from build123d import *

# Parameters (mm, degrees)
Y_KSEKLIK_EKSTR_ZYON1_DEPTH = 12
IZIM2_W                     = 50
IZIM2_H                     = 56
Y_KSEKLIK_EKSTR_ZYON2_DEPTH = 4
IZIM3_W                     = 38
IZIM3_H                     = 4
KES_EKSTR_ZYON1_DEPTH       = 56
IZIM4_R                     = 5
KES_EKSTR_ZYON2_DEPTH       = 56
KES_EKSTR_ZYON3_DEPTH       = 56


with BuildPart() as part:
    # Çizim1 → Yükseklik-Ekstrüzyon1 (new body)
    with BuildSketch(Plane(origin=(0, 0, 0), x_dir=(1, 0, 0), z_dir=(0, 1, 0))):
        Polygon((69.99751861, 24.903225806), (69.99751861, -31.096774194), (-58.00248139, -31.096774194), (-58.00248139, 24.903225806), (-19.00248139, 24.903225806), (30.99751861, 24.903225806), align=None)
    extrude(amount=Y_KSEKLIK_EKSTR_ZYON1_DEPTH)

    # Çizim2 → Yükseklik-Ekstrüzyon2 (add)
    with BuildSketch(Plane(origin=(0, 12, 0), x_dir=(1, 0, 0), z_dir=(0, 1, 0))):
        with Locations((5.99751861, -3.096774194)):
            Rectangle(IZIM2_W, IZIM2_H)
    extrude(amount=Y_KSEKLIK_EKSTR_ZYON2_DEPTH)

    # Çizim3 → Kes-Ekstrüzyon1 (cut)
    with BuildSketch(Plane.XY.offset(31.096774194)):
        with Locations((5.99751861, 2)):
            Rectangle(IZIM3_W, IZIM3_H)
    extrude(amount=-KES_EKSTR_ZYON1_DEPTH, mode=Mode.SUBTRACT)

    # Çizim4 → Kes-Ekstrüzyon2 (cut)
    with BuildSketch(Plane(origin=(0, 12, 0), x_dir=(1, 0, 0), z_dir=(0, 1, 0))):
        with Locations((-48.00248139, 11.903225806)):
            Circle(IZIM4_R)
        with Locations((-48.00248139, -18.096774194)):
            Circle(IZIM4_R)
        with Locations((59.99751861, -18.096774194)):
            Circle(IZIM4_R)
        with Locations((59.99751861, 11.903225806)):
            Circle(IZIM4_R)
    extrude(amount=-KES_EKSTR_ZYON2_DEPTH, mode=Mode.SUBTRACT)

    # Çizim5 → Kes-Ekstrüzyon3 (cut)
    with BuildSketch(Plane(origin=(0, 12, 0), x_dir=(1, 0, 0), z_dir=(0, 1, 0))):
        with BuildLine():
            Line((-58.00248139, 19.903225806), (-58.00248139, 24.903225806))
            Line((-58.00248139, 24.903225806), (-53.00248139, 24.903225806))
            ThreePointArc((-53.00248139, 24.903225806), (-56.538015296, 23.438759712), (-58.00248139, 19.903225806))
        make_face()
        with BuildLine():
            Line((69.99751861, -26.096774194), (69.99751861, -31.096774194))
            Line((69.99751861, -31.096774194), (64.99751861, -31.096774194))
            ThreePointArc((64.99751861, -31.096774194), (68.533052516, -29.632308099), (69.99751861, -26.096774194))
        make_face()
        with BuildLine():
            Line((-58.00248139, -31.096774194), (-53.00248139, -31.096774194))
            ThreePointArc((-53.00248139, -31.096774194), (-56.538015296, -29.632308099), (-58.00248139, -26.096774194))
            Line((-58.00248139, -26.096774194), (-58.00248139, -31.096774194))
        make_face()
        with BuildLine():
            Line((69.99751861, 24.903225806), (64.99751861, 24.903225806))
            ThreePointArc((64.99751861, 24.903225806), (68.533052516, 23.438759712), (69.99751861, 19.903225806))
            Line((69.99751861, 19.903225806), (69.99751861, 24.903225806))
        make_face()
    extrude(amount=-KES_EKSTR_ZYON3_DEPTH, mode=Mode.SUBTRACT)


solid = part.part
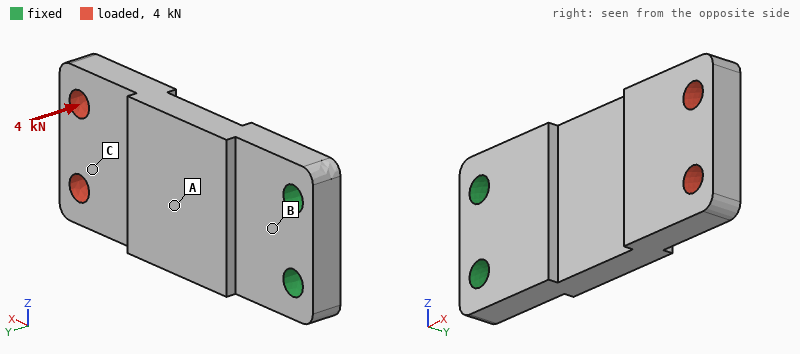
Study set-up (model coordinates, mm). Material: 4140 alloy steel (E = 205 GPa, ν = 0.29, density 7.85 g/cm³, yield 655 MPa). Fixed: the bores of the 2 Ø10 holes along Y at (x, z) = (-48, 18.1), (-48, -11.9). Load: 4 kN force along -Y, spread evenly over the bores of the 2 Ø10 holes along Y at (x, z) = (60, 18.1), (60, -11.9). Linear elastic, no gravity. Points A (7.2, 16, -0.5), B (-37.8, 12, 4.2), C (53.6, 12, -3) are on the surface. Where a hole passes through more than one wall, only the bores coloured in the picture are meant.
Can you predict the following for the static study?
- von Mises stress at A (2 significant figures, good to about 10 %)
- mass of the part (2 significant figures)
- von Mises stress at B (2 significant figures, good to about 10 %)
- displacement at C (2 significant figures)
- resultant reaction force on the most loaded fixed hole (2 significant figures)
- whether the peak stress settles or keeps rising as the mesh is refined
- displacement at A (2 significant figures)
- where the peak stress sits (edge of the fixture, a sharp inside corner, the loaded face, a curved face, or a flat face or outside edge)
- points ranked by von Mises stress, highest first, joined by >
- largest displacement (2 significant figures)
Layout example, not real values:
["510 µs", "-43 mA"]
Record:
["150 MPa", "660 g", "230 MPa", "0.89 mm", "2.0 kN", "keeps rising", "0.32 mm", "edge of the fixture", "B > A > C", "1.1 mm"]
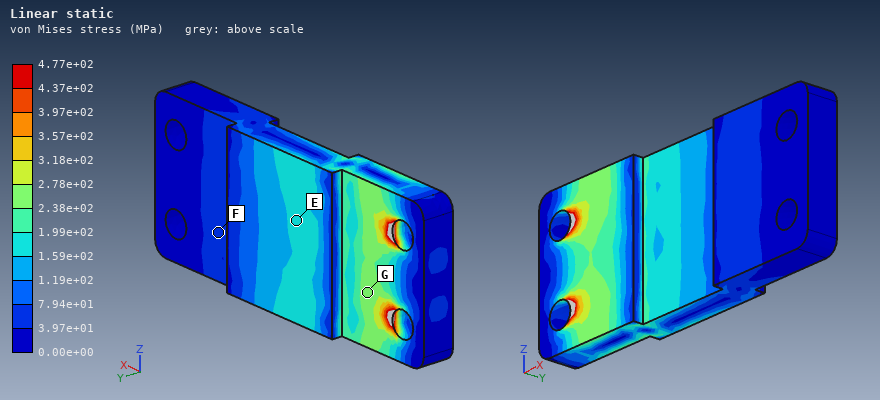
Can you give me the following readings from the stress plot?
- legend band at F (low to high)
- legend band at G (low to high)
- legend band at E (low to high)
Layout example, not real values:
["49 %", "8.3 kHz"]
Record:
["3.97e+01 to 7.94e+01 MPa", "2.38e+02 to 2.78e+02 MPa", "1.59e+02 to 1.99e+02 MPa"]
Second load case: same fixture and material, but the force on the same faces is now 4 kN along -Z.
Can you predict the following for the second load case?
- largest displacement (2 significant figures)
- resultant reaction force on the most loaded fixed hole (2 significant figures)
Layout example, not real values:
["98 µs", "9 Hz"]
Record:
["80 µm", "12 kN"]
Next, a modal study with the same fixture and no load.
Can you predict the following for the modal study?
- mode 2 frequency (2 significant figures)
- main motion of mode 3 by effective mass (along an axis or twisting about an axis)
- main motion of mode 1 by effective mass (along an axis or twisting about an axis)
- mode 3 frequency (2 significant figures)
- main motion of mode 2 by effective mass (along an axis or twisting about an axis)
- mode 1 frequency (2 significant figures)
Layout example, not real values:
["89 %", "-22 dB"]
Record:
["2600 Hz", "along Z", "along Y", "3200 Hz", "along Z", "750 Hz"]
